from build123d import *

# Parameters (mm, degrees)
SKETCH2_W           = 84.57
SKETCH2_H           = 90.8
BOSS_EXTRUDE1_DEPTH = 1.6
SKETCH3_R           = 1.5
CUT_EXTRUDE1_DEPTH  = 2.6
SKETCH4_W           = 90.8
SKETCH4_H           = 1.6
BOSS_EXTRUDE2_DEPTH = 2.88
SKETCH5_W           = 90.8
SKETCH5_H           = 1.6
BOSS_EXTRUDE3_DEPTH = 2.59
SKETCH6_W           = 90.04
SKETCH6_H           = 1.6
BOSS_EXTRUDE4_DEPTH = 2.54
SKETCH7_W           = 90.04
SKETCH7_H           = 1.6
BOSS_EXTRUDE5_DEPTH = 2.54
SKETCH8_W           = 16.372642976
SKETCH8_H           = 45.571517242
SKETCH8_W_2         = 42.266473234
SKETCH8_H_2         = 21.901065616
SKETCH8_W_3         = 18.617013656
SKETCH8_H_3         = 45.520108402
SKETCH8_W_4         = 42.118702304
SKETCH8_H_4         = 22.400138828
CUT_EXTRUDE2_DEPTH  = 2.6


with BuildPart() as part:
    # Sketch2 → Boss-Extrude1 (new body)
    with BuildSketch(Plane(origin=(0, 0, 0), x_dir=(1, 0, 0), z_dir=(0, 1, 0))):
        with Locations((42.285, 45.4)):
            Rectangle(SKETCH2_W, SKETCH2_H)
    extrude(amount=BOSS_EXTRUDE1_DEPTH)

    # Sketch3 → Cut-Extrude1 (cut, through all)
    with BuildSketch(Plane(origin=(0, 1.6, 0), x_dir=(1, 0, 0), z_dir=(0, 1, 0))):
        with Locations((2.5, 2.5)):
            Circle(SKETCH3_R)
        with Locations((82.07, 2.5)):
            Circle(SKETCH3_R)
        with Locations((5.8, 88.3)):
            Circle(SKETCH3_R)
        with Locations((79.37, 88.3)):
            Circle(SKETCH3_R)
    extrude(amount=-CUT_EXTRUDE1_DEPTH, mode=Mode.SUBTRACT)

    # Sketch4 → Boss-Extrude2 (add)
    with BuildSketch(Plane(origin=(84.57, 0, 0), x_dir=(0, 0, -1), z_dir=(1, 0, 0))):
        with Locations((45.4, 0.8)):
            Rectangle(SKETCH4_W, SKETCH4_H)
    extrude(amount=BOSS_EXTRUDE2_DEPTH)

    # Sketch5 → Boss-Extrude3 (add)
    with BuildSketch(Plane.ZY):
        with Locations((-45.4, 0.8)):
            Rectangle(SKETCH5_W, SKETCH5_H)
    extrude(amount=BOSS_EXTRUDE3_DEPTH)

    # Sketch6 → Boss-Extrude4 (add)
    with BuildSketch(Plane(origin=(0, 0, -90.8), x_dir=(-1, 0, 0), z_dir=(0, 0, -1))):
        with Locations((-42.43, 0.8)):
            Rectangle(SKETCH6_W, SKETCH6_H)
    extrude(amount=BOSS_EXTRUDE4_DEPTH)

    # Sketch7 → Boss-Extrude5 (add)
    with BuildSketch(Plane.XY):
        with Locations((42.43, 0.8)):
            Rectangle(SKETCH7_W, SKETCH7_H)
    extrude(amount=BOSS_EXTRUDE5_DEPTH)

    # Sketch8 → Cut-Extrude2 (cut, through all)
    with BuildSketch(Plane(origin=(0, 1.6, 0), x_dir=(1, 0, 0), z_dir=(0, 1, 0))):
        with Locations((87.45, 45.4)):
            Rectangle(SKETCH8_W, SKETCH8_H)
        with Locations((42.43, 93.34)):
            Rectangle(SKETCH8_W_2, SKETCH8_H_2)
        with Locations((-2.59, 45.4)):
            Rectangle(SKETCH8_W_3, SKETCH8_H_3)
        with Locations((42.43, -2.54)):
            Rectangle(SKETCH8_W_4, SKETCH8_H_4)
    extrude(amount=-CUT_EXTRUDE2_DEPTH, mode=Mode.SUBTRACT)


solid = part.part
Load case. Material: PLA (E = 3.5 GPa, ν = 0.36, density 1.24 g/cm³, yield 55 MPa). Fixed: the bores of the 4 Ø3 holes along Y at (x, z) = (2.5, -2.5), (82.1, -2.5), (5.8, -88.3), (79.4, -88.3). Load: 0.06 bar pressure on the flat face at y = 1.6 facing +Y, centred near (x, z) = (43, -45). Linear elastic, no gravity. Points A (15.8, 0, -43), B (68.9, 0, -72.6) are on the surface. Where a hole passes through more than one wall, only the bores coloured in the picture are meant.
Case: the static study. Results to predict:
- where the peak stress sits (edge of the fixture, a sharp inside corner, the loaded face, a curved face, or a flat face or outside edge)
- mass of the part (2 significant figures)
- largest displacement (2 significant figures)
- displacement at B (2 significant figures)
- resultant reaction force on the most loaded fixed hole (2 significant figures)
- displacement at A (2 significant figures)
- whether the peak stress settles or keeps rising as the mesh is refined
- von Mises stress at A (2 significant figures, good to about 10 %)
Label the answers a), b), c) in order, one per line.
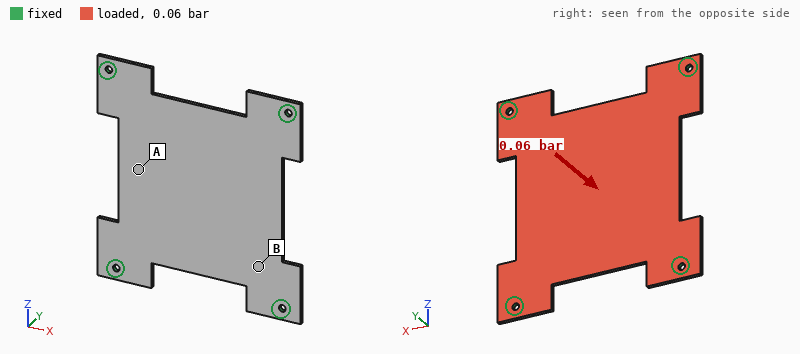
a) edge of the fixture
b) 14 g
c) 1.5 mm
d) 0.61 mm
e) 10 N
f) 1.2 mm
g) keeps rising
h) 5.4 MPa
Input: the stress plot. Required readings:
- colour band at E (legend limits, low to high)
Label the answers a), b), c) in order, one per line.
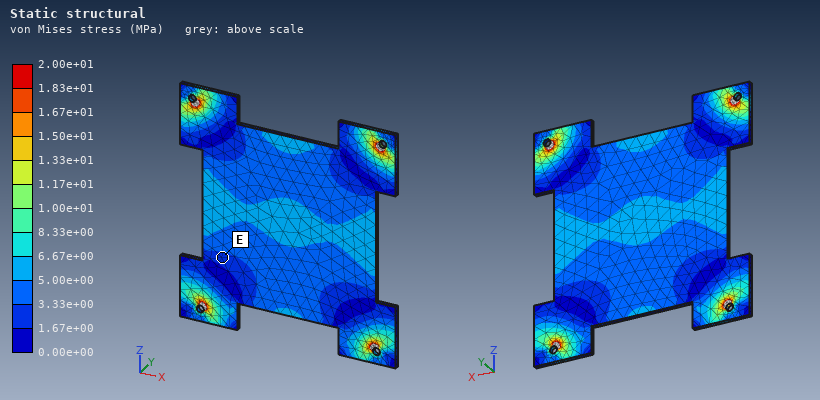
a) 1.67e+00 to 3.33e+00 MPa
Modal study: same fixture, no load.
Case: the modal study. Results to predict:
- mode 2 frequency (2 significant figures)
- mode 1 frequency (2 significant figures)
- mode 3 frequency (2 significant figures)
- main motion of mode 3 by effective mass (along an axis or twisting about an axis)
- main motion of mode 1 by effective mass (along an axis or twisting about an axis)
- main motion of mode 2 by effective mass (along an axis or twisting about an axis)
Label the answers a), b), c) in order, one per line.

a) 480 Hz
b) 260 Hz
c) 540 Hz
d) twisting about X
e) along Y
f) twisting about Z
